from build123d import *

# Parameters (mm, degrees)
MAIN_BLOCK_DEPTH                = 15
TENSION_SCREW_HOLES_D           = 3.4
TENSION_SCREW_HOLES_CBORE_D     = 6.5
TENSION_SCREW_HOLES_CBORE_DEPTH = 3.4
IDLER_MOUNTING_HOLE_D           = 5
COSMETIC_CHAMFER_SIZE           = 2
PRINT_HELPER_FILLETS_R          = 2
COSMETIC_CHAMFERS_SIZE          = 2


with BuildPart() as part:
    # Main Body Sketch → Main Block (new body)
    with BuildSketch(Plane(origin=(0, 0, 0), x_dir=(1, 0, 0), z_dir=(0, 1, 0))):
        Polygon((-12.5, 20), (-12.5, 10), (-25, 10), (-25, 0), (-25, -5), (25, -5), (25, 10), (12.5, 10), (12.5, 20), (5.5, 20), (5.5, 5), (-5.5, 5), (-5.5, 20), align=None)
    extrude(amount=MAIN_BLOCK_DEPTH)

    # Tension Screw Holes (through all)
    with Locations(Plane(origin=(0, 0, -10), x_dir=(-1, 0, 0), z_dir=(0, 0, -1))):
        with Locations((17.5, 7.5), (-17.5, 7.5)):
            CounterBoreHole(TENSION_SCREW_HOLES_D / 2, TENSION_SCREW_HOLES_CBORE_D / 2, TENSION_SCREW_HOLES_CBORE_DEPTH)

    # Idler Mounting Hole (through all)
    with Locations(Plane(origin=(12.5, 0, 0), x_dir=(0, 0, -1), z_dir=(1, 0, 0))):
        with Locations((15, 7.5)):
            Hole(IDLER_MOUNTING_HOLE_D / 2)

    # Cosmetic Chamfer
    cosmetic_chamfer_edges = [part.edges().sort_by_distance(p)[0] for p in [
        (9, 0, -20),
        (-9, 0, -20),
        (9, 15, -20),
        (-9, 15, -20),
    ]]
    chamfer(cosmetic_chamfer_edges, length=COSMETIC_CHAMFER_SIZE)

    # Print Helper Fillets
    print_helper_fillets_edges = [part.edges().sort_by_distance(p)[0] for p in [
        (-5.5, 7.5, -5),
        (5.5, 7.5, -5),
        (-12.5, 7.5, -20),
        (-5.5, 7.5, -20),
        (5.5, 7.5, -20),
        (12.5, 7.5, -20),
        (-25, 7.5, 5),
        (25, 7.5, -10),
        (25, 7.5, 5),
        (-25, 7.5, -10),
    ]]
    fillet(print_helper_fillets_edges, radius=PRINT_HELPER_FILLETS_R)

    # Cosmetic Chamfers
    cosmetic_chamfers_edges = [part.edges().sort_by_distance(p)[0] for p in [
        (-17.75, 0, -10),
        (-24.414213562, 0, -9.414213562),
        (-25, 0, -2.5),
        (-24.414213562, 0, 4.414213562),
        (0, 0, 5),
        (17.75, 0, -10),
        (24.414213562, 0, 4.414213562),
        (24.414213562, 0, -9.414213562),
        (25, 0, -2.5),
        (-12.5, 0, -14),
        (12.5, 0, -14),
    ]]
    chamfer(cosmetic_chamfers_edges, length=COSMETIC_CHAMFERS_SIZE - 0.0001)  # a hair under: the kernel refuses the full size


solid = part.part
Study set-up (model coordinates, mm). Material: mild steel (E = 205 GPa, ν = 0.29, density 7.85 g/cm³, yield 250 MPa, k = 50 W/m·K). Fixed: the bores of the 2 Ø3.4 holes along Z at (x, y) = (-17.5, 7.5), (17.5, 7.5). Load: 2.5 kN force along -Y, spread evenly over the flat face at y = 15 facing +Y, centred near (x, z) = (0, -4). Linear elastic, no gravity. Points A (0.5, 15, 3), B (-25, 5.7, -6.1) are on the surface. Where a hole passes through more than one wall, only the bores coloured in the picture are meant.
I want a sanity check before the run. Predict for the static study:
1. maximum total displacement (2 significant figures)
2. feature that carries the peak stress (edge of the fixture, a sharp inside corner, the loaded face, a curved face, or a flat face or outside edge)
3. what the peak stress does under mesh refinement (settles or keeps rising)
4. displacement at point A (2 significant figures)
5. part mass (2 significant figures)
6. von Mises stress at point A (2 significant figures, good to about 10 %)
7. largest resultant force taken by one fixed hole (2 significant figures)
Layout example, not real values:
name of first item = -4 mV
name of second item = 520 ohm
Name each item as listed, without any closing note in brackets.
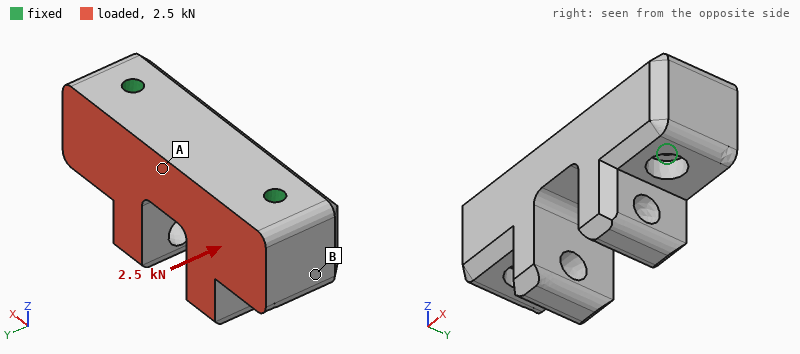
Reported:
maximum total displacement = 2.8 µm
feature that carries the peak stress = edge of the fixture
what the peak stress does under mesh refinement = keeps rising
displacement at point A = 1.1 µm
part mass = 90 g
von Mises stress at point A = 9.7 MPa
largest resultant force taken by one fixed hole = 1.3 kN
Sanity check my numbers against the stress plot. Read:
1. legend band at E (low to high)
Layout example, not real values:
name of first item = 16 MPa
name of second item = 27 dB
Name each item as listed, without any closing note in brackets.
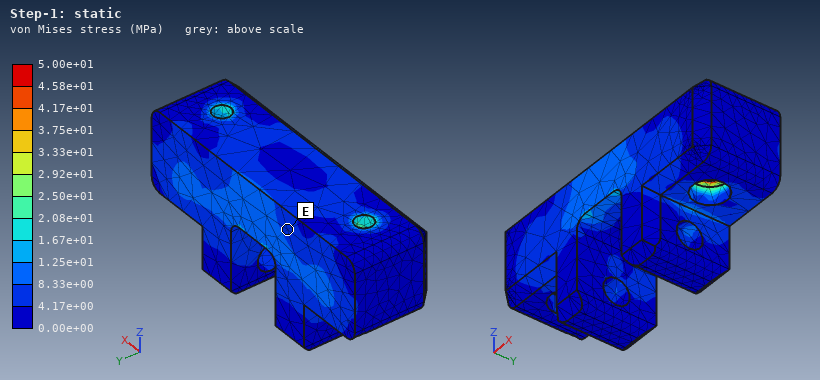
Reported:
legend band at E = 4.17e+00 to 8.33e+00 MPa
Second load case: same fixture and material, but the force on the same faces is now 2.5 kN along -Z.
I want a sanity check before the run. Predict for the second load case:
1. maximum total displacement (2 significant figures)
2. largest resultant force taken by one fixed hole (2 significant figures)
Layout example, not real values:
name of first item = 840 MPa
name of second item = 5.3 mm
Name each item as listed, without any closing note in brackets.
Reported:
maximum total displacement = 4.1 µm
largest resultant force taken by one fixed hole = 1.3 kN
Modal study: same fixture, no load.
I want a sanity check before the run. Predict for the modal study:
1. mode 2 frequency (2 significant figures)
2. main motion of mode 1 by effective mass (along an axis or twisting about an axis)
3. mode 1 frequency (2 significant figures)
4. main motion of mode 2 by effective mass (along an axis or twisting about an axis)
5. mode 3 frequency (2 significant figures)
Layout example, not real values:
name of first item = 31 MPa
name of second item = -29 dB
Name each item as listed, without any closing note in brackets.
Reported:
mode 2 frequency = 20 kHz
main motion of mode 1 by effective mass = along Y
mode 1 frequency = 19 kHz
main motion of mode 2 by effective mass = along Z
mode 3 frequency = 24 kHz
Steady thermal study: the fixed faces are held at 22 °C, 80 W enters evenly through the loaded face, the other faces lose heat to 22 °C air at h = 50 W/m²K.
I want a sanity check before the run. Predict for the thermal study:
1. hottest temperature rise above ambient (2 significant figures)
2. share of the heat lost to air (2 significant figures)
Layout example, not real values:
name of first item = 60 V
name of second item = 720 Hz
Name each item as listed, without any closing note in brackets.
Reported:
hottest temperature rise above ambient = 40 K
share of the heat lost to air = 4.3 %
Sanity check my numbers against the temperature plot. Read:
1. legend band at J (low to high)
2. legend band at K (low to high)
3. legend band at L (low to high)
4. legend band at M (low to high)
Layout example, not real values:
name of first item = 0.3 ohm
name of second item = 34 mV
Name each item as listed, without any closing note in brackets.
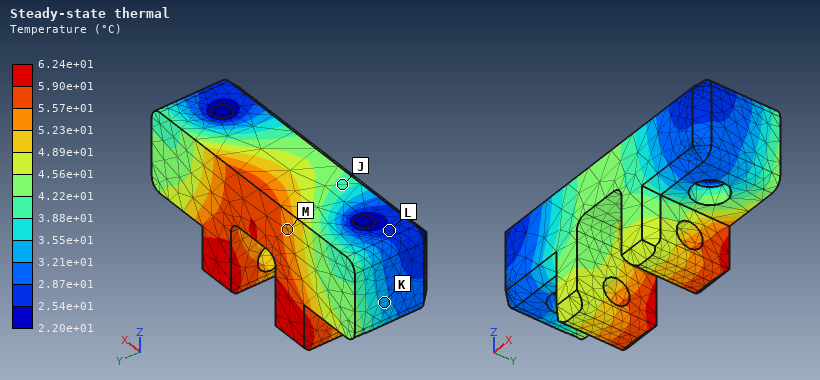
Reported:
legend band at J = 3.88e+01 to 4.22e+01 °C
legend band at K = 3.21e+01 to 3.55e+01 °C
legend band at L = 2.54e+01 to 2.87e+01 °C
legend band at M = 5.23e+01 to 5.57e+01 °C
